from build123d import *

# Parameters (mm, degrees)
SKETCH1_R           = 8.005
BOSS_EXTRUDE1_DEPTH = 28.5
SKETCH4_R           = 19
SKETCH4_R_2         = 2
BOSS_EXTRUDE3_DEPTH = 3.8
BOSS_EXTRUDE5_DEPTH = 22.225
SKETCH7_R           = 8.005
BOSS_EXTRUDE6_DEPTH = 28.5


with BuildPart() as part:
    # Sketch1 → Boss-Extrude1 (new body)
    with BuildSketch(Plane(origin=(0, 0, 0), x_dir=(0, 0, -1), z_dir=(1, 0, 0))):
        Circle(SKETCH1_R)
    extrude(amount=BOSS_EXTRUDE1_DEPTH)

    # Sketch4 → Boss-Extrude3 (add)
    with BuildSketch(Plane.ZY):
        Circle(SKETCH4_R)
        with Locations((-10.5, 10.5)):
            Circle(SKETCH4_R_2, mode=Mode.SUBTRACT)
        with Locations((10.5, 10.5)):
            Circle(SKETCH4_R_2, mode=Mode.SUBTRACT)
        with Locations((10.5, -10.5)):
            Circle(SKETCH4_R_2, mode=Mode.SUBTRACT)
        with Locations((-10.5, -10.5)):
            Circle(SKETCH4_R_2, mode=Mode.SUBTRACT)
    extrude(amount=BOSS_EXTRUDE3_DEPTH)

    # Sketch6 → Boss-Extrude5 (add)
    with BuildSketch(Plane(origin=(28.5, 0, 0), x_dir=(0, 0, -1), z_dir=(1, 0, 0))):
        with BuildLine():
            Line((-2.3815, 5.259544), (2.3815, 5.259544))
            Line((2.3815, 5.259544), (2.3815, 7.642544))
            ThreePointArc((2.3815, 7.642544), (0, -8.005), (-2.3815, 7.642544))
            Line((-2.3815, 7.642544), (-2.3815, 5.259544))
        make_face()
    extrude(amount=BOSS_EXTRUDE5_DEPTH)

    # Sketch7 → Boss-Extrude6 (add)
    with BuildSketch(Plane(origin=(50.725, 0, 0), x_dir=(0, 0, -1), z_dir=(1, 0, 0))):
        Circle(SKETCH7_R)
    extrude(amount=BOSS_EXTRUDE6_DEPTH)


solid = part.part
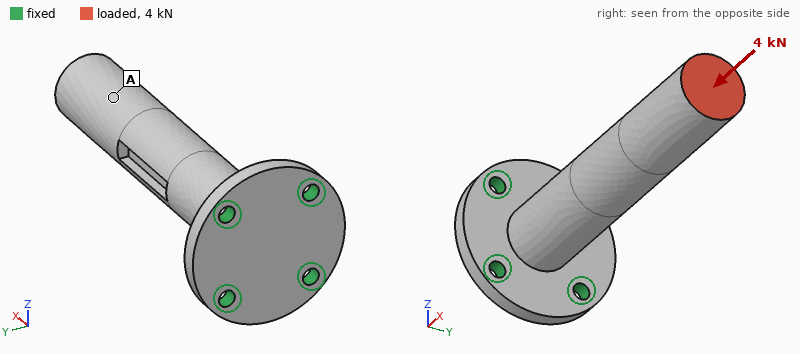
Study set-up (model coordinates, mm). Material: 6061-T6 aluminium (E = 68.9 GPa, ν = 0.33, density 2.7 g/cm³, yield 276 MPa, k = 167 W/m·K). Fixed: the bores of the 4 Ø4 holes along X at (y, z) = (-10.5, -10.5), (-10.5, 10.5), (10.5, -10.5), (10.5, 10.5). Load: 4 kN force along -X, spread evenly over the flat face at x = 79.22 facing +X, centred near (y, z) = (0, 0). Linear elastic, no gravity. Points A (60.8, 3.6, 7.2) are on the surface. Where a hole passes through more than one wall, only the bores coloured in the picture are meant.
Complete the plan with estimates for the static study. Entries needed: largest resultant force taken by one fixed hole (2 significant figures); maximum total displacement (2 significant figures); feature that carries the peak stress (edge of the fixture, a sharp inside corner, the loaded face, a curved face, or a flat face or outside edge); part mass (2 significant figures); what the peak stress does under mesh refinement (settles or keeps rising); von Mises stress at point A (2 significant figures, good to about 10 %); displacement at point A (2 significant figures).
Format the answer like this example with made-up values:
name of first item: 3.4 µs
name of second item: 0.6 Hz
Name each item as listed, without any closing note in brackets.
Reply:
largest resultant force taken by one fixed hole: 1.0 kN
maximum total displacement: 43 µm
feature that carries the peak stress: edge of the fixture
part mass: 53 g
what the peak stress does under mesh refinement: keeps rising
von Mises stress at point A: 20 MPa
displacement at point A: 36 µm
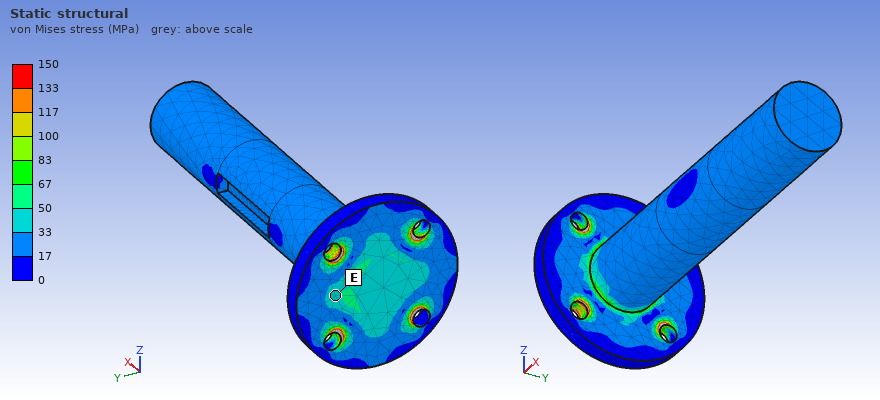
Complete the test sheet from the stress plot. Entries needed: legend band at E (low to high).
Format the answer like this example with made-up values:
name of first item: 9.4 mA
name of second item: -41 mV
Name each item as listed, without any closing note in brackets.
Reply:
legend band at E: 33 to 50 MPa
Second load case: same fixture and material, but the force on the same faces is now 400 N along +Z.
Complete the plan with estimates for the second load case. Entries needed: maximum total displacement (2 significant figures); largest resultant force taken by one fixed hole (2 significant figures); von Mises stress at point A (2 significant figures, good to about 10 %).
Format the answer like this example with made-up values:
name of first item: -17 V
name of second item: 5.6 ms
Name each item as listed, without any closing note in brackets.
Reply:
maximum total displacement: 0.47 mm
largest resultant force taken by one fixed hole: 900 N
von Mises stress at point A: 17 MPa
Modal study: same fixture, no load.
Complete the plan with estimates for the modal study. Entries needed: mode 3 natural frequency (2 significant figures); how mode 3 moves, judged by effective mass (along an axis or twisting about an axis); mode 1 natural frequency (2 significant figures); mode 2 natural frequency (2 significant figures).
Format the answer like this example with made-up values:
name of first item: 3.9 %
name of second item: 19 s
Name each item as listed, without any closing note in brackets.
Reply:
mode 3 natural frequency: 8000 Hz
how mode 3 moves, judged by effective mass: along Y
mode 1 natural frequency: 1300 Hz
mode 2 natural frequency: 1400 Hz
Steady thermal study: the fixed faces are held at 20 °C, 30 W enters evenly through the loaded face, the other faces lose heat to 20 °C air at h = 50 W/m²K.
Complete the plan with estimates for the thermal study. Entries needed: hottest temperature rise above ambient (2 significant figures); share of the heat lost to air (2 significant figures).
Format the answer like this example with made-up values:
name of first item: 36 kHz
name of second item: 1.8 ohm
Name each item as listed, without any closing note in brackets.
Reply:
hottest temperature rise above ambient: 67 K
share of the heat lost to air: 25 %
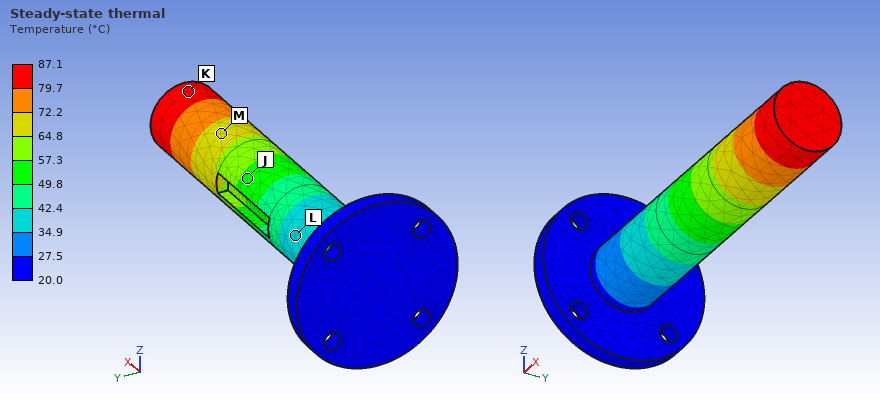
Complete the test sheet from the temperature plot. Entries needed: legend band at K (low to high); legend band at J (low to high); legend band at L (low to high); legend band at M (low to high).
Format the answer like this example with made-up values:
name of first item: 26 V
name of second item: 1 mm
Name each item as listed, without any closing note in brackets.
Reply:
legend band at K: 79.7 to 87.1 °C
legend band at J: 49.8 to 57.3 °C
legend band at L: 34.9 to 42.4 °C
legend band at M: 64.8 to 72.2 °C
